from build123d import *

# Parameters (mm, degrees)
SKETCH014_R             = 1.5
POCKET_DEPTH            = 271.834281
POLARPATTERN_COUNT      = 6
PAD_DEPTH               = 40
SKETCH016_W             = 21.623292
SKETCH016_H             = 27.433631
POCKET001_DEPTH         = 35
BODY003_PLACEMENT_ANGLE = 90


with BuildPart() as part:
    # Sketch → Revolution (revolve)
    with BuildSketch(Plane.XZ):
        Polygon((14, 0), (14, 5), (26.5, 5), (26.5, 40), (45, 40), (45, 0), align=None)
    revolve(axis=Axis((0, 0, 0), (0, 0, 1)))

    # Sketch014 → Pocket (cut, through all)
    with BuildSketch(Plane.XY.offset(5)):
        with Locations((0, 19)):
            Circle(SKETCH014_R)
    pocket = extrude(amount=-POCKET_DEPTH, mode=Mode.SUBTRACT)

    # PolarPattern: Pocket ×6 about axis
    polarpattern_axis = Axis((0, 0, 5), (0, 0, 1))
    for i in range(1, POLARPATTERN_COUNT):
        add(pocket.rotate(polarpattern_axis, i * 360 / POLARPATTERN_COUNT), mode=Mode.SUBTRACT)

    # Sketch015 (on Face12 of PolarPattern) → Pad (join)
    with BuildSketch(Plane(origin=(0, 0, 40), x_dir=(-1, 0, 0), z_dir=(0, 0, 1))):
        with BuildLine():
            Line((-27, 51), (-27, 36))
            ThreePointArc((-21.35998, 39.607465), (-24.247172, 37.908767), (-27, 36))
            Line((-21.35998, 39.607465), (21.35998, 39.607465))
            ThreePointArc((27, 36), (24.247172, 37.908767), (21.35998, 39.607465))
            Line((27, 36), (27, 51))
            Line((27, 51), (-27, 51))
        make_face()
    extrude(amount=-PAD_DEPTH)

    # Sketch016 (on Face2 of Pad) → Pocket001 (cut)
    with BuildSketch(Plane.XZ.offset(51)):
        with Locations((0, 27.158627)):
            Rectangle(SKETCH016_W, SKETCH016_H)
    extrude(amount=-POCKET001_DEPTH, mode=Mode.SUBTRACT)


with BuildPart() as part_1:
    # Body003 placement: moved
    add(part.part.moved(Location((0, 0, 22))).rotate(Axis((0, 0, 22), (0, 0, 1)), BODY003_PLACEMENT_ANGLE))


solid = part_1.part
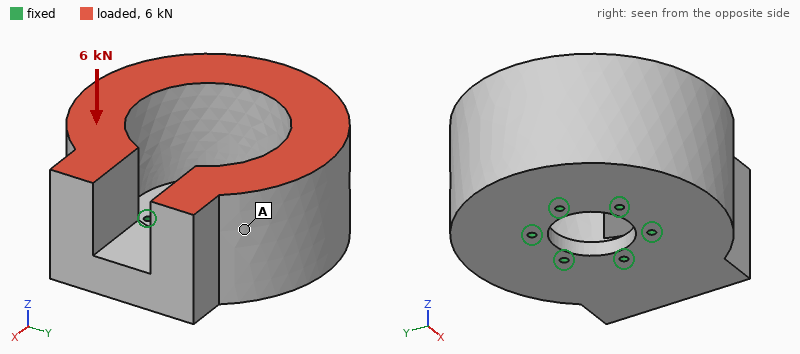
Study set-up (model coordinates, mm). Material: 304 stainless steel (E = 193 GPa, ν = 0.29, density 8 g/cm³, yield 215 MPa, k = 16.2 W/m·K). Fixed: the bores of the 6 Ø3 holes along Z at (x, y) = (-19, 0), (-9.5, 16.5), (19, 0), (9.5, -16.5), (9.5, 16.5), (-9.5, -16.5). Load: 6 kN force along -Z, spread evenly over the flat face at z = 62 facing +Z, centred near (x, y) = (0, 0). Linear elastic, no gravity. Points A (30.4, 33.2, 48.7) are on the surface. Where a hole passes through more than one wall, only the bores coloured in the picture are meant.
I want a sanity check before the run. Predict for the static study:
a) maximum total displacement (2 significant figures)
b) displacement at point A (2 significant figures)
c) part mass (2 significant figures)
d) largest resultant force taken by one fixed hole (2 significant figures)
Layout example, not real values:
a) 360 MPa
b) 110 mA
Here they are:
a) 8.9 µm
b) 7.1 µm
c) 1.4 kg
d) 1.2 kN
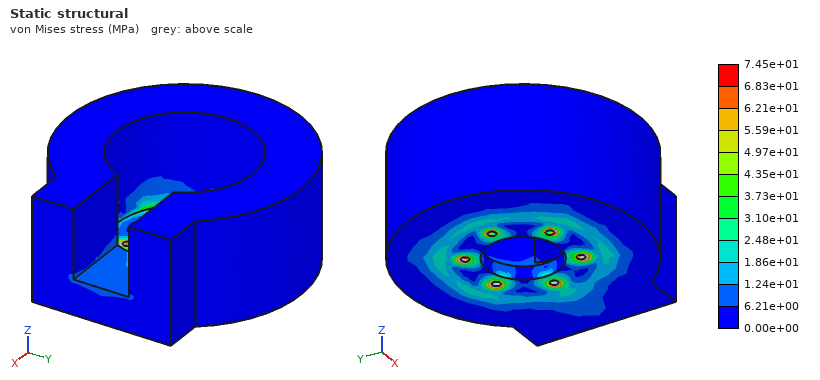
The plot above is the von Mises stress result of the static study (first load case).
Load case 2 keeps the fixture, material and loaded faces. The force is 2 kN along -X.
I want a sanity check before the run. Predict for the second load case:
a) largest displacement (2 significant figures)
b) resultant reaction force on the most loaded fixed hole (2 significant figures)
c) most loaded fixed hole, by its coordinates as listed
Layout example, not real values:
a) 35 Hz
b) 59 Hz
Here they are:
a) 19 µm
b) 1.1 kN
c) (-19, 0)
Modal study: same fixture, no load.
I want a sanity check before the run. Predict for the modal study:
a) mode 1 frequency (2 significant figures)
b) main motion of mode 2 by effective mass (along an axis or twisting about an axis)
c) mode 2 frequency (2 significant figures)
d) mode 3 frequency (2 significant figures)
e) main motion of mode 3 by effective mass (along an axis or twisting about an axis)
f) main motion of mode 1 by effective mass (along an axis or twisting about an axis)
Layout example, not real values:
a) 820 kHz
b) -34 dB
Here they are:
a) 2100 Hz
b) along Y
c) 2300 Hz
d) 4700 Hz
e) along Z
f) along X
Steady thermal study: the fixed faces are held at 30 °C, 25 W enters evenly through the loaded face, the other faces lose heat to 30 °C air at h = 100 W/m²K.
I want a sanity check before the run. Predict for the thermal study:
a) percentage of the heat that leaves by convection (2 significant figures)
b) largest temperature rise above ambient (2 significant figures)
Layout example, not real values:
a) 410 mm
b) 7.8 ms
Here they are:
a) 81 %
b) 15 K
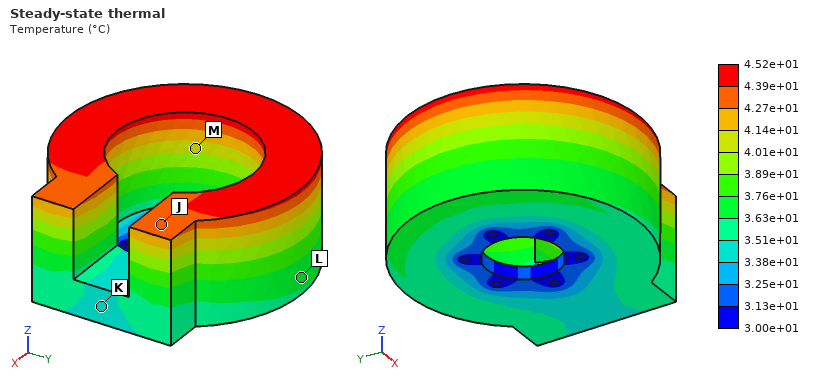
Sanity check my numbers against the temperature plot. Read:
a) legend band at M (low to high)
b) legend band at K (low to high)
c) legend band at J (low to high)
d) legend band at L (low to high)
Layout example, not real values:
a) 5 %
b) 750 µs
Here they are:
a) 4.01e+01 to 4.14e+01 °C
b) 3.38e+01 to 3.51e+01 °C
c) 4.27e+01 to 4.39e+01 °C
d) 3.63e+01 to 3.76e+01 °C
